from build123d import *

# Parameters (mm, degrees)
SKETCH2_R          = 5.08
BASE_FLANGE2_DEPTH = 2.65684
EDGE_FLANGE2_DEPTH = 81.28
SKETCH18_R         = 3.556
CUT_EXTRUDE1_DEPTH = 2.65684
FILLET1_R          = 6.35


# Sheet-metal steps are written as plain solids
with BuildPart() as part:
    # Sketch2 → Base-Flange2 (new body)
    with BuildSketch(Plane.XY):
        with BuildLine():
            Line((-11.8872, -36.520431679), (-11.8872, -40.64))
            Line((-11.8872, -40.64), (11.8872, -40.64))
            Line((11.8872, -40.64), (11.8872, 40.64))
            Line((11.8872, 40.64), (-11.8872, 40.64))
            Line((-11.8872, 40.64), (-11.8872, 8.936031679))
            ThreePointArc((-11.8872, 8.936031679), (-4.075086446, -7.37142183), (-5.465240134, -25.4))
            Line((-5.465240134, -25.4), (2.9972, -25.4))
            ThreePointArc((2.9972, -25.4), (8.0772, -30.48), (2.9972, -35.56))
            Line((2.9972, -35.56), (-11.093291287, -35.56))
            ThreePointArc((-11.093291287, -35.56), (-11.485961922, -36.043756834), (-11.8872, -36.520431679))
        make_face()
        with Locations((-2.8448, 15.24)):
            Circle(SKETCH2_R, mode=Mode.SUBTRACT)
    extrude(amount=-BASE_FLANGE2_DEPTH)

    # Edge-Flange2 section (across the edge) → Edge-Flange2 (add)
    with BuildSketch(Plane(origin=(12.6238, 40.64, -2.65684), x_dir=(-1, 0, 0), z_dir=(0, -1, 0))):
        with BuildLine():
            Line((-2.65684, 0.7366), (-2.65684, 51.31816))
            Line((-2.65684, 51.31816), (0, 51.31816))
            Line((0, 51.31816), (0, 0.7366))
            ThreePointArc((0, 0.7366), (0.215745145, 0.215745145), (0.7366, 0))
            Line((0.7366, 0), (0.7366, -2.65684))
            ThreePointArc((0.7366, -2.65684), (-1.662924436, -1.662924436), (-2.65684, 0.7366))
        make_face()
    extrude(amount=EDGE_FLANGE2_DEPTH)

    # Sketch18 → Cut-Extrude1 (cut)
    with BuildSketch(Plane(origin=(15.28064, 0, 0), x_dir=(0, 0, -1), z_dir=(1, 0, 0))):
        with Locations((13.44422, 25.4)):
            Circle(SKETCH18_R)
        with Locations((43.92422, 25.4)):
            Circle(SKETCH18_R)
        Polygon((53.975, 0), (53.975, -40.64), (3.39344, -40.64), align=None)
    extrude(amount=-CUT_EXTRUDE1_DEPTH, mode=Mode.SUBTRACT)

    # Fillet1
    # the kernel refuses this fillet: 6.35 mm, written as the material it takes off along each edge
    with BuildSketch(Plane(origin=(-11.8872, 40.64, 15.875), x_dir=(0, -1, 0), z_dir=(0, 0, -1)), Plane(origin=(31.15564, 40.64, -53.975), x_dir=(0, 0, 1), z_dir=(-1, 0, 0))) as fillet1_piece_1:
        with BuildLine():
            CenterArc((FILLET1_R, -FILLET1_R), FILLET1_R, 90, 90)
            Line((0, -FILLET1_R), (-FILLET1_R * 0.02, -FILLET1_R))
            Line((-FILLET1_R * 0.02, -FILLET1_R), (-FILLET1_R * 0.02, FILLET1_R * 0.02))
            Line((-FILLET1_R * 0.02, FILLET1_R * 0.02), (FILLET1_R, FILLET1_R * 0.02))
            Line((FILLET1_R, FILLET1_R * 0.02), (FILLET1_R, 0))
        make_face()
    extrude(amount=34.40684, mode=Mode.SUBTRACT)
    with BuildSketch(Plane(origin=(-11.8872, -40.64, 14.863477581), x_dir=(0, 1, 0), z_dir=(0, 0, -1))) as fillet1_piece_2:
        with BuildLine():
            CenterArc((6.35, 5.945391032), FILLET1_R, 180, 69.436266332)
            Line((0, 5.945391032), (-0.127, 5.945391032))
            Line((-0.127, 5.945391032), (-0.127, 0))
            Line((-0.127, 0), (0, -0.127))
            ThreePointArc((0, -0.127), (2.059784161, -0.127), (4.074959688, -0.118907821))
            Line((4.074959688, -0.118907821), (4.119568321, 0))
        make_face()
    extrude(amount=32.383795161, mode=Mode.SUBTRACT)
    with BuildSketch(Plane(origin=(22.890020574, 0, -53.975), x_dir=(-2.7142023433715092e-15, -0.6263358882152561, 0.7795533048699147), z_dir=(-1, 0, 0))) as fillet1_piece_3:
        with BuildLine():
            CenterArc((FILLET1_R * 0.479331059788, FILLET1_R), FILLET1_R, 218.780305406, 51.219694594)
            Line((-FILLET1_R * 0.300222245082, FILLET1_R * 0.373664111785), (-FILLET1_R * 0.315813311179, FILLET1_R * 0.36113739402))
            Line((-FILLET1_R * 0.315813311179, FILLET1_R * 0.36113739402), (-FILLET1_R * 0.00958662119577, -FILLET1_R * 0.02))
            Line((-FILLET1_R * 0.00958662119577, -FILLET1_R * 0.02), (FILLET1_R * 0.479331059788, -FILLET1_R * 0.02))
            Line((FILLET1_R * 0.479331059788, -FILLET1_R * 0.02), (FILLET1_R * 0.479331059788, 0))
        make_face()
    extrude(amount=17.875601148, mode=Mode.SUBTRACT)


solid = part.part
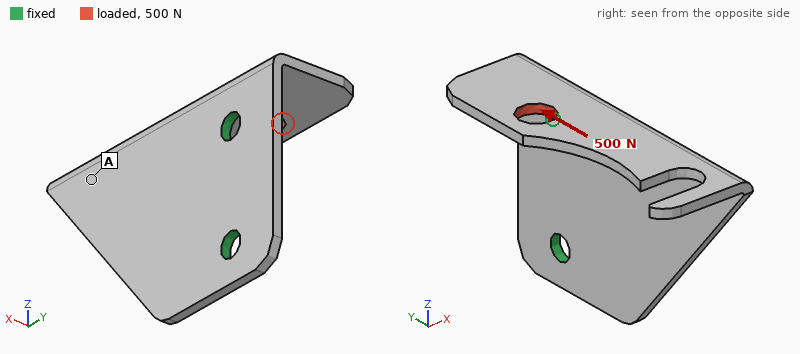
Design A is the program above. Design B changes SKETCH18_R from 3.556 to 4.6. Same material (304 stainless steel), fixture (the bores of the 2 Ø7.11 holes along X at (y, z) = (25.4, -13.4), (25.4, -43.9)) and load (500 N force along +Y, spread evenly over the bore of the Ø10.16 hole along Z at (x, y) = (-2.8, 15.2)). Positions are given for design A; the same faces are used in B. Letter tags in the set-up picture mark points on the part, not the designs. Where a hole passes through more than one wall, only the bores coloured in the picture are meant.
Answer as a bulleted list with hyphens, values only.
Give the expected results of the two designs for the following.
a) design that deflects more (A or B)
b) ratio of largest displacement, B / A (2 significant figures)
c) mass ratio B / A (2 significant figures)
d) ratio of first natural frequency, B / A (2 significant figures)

- A
- 0.81
- 0.99
- 1.1
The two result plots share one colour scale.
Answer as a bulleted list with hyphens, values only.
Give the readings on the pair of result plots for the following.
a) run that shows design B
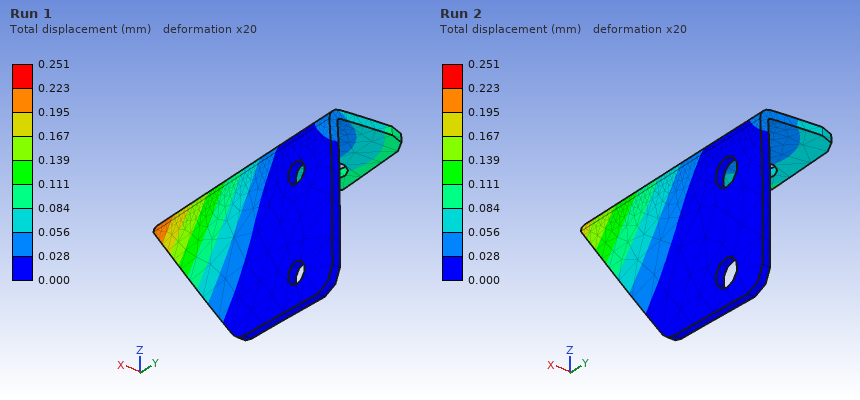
- Run 2
